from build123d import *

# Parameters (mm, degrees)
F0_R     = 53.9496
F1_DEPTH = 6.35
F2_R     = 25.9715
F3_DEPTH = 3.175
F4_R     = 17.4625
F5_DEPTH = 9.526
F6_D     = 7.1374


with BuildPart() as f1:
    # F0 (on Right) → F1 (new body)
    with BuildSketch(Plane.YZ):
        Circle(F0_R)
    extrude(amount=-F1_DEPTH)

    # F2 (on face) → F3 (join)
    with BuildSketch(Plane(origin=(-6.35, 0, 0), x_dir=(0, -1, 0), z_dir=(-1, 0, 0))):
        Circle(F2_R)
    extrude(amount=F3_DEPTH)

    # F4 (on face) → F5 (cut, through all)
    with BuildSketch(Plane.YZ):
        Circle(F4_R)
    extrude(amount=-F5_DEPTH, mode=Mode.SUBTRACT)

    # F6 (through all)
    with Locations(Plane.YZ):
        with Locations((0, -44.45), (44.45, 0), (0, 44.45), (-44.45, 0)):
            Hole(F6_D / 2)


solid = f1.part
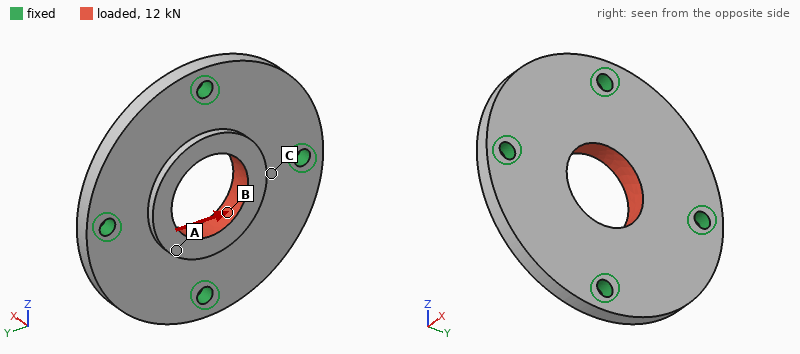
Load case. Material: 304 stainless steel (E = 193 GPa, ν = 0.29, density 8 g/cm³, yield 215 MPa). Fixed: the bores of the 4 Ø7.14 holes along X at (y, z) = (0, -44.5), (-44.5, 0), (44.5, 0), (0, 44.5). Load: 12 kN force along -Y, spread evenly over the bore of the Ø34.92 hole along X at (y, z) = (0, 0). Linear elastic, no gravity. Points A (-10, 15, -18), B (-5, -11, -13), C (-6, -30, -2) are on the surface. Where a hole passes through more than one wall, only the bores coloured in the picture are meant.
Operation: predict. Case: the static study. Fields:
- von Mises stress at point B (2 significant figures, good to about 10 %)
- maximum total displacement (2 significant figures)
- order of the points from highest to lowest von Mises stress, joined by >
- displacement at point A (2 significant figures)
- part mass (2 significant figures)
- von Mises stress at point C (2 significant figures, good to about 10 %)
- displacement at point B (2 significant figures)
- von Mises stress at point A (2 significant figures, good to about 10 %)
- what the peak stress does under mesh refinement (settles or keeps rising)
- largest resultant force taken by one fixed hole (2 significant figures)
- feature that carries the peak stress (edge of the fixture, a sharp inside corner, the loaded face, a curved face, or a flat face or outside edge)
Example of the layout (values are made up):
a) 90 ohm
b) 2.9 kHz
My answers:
a) 18 MPa
b) 4.3 µm
c) C > B > A
d) 3.8 µm
e) 440 g
f) 34 MPa
g) 3.9 µm
h) 7.0 MPa
i) keeps rising
j) 3.6 kN
k) edge of the fixture
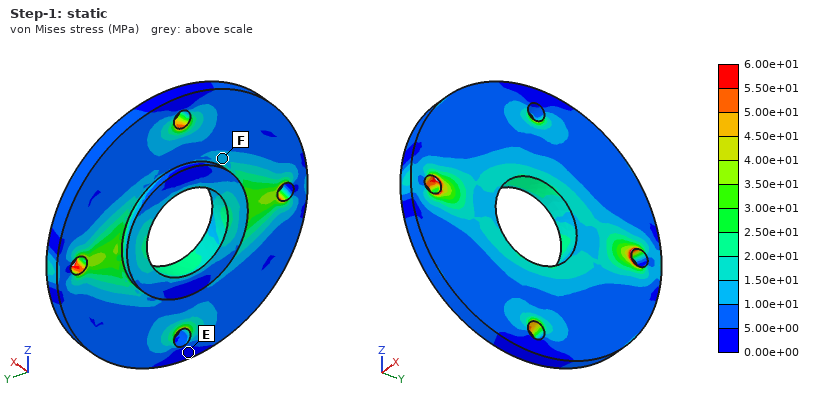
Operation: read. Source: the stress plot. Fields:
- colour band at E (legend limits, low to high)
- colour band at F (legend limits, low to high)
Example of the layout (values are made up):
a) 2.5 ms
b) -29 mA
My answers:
a) 0.00e+00 to 5.00e+00 MPa
b) 1.00e+01 to 1.50e+01 MPa
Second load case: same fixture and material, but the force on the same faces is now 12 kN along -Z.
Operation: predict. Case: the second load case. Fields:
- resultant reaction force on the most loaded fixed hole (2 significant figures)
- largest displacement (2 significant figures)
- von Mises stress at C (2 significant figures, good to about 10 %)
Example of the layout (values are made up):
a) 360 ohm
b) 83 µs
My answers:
a) 3.6 kN
b) 4.3 µm
c) 8.0 MPa
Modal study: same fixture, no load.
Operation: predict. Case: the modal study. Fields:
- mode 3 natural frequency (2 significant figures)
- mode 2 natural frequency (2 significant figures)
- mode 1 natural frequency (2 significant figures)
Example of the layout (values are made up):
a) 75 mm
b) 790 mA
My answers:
a) 6700 Hz
b) 6700 Hz
c) 6400 Hz
